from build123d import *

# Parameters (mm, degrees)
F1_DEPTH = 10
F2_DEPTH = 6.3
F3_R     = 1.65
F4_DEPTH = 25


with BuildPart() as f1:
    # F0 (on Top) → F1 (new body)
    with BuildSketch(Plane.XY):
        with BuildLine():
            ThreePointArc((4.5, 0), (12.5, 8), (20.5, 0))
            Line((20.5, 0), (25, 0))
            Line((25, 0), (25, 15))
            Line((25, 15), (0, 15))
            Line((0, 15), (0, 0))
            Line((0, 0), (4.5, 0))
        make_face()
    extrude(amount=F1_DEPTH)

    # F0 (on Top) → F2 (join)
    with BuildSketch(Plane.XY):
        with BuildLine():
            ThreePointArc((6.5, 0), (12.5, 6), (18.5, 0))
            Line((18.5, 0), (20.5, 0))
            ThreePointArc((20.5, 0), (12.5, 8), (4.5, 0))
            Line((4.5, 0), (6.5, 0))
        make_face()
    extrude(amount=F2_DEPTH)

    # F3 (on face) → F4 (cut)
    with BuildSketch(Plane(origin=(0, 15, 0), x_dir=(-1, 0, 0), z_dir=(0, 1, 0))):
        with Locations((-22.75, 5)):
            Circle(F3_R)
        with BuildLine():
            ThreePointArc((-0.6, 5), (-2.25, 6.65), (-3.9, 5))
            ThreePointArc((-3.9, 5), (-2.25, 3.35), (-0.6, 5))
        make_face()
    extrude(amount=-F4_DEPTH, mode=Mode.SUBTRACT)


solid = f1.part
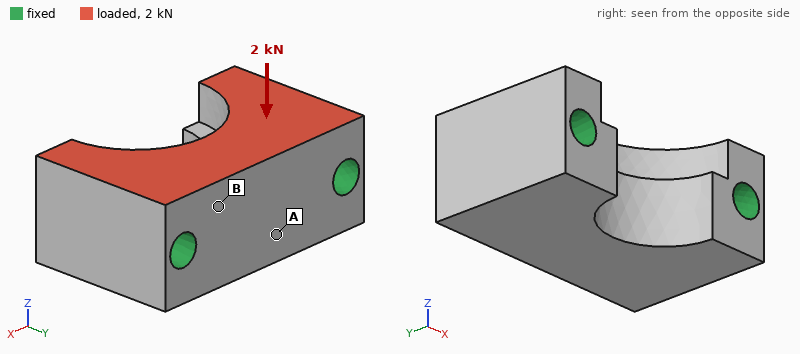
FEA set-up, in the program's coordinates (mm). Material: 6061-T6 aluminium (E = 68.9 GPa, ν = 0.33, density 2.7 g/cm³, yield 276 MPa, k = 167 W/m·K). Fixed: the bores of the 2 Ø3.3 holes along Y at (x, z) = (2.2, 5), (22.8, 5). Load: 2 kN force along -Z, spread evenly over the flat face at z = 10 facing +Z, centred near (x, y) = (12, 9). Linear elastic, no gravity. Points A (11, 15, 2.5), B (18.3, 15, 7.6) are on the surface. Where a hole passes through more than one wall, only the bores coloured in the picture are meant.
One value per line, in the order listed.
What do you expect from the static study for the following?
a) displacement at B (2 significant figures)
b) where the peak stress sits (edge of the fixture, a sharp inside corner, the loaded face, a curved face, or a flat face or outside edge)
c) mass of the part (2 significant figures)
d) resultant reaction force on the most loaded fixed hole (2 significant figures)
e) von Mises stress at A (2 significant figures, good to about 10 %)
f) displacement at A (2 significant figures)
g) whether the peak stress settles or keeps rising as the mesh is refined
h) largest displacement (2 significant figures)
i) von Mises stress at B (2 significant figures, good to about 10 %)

1.6 µm
edge of the fixture
7.5 g
1.0 kN
4.9 MPa
2.3 µm
keeps rising
2.9 µm
11 MPa
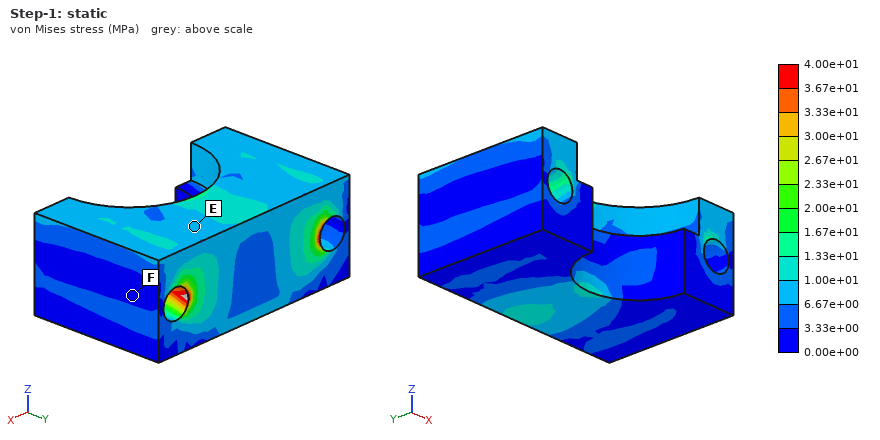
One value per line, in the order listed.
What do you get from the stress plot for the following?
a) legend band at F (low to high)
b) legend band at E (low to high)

0.00e+00 to 3.33e+00 MPa
6.67e+00 to 1.00e+01 MPa
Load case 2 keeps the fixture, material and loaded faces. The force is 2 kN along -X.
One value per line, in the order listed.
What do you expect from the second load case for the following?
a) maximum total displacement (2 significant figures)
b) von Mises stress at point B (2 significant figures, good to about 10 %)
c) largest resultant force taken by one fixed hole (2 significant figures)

2.8 µm
14 MPa
1.0 kN
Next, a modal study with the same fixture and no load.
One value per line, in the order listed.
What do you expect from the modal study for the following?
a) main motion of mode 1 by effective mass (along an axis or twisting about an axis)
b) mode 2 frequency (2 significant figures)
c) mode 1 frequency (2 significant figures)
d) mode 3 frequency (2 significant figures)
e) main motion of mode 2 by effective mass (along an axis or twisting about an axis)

along Z
75 kHz
59 kHz
89 kHz
along Y
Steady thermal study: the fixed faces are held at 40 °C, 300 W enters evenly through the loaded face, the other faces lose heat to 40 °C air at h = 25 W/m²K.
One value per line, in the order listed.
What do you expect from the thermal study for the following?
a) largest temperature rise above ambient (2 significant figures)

51 K
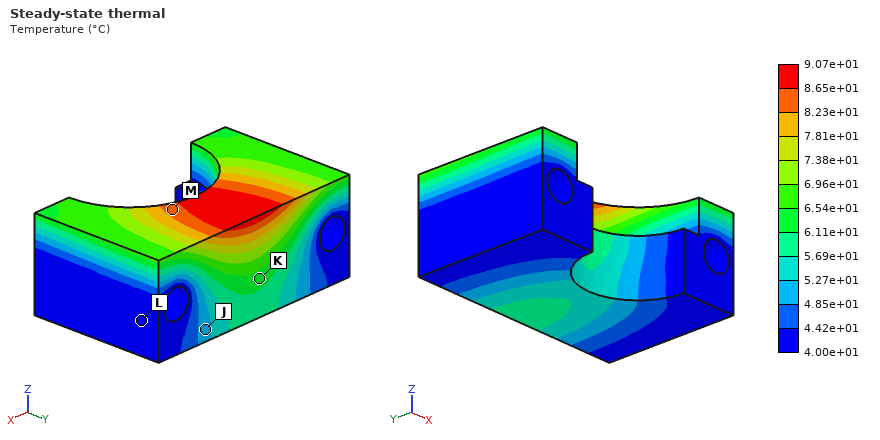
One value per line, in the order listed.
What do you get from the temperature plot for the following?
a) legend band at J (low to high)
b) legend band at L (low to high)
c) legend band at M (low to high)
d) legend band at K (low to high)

4.85e+01 to 5.27e+01 °C
4.00e+01 to 4.42e+01 °C
8.23e+01 to 8.65e+01 °C
6.11e+01 to 6.54e+01 °C
